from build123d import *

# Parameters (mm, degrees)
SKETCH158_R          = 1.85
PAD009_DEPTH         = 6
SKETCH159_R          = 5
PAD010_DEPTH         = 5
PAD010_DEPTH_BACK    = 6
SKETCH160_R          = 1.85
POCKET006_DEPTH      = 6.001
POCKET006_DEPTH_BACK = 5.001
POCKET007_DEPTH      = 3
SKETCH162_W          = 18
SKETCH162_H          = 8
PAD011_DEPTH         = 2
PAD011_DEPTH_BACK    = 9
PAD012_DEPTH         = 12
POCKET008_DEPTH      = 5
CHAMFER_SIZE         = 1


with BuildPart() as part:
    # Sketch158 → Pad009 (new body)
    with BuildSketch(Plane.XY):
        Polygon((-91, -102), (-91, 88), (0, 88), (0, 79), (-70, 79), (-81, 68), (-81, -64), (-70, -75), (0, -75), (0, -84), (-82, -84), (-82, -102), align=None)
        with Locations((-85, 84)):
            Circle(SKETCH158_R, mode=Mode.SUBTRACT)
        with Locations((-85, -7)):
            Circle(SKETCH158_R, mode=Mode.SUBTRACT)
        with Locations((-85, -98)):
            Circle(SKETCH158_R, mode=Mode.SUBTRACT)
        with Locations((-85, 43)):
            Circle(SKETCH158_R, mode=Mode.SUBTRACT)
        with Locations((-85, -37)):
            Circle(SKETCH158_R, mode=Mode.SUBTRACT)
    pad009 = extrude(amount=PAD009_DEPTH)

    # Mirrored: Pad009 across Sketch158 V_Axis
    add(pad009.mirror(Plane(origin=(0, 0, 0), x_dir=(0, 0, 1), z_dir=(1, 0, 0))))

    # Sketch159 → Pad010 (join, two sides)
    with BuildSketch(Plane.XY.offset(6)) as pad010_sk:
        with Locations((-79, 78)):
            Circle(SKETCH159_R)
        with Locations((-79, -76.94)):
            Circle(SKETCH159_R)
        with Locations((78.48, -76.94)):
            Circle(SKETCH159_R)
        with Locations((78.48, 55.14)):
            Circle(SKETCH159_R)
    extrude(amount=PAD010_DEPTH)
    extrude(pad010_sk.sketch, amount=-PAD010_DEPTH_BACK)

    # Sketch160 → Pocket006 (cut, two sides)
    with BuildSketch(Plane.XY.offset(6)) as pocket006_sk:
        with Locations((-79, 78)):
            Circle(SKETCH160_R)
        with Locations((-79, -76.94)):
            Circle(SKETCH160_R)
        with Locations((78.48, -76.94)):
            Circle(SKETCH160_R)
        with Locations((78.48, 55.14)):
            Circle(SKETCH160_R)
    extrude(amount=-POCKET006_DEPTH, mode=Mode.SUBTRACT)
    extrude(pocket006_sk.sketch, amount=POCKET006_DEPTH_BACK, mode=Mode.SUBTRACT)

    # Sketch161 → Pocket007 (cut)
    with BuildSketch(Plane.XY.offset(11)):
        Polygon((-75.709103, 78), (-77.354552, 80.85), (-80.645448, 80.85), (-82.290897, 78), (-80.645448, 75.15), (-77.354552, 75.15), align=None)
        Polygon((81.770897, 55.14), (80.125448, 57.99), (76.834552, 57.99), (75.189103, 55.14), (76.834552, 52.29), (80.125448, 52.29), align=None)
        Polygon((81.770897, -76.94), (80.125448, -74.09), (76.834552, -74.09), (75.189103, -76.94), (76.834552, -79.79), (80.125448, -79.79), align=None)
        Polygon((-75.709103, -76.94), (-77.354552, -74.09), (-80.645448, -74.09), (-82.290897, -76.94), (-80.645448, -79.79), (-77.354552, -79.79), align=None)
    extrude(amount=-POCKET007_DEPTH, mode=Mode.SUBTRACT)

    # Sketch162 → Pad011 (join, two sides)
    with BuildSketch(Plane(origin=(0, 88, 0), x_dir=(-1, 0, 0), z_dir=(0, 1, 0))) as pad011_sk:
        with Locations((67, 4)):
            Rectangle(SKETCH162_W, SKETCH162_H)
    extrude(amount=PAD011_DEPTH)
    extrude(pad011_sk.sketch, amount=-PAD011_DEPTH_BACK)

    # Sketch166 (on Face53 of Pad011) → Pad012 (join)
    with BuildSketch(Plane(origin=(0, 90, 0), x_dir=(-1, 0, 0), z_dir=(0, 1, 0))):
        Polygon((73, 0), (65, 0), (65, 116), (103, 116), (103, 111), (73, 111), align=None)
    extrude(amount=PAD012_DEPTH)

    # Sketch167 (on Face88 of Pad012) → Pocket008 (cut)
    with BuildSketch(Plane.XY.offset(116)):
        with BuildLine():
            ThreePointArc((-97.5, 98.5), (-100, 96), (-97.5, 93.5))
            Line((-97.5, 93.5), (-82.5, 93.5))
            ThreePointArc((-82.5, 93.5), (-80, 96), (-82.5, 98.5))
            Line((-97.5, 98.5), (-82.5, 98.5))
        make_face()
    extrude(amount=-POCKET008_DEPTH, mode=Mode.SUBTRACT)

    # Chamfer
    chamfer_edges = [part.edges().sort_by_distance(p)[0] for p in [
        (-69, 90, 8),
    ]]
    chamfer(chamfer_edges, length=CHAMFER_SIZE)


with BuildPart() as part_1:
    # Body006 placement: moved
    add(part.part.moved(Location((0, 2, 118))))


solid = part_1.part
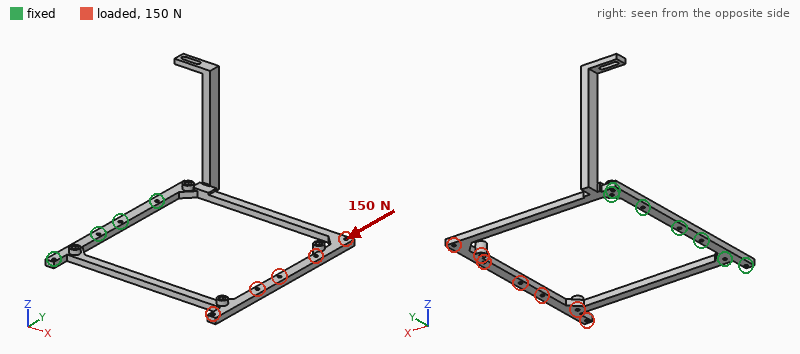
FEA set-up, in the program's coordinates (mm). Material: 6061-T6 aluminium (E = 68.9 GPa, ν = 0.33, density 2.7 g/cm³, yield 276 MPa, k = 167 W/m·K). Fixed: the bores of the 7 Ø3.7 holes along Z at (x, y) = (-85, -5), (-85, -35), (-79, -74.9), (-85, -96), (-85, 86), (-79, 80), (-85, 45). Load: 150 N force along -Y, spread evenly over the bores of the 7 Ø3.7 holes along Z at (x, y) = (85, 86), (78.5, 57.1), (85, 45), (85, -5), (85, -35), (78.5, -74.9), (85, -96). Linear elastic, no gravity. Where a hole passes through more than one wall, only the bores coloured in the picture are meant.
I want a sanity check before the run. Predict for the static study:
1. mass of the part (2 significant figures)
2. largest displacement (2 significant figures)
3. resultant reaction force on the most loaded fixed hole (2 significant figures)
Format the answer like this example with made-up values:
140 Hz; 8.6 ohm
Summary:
150 g; 1.1 mm; 710 N
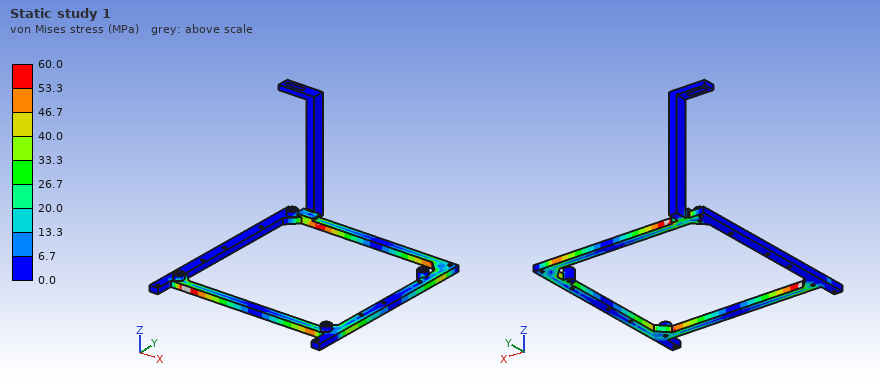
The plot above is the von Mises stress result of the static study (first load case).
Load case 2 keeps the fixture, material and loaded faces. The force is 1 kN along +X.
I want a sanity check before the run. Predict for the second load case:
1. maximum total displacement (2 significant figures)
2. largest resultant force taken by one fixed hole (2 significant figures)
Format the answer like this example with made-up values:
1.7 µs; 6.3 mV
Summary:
0.51 mm; 550 N
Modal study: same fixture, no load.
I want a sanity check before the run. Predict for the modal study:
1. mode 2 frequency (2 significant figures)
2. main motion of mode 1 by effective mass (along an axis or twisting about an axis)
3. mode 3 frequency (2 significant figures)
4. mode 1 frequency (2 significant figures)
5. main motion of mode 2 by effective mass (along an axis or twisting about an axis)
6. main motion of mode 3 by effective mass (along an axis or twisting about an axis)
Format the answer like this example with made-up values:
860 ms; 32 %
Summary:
220 Hz; along Z; 270 Hz; 99 Hz; twisting about X; along Y
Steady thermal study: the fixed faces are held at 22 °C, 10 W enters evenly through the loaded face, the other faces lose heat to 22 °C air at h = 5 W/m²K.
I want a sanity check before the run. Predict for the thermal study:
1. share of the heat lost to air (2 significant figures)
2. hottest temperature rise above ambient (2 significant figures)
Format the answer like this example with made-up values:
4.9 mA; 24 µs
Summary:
35 %; 67 K
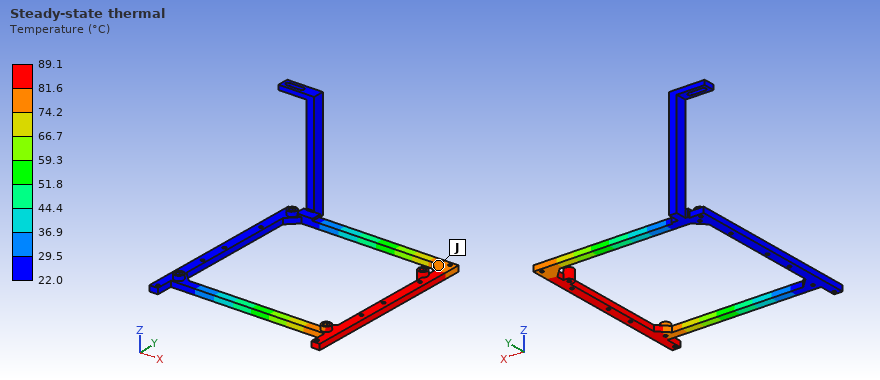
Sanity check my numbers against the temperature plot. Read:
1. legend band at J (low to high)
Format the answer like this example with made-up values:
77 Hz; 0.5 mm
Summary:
74.2 to 81.6 °C
